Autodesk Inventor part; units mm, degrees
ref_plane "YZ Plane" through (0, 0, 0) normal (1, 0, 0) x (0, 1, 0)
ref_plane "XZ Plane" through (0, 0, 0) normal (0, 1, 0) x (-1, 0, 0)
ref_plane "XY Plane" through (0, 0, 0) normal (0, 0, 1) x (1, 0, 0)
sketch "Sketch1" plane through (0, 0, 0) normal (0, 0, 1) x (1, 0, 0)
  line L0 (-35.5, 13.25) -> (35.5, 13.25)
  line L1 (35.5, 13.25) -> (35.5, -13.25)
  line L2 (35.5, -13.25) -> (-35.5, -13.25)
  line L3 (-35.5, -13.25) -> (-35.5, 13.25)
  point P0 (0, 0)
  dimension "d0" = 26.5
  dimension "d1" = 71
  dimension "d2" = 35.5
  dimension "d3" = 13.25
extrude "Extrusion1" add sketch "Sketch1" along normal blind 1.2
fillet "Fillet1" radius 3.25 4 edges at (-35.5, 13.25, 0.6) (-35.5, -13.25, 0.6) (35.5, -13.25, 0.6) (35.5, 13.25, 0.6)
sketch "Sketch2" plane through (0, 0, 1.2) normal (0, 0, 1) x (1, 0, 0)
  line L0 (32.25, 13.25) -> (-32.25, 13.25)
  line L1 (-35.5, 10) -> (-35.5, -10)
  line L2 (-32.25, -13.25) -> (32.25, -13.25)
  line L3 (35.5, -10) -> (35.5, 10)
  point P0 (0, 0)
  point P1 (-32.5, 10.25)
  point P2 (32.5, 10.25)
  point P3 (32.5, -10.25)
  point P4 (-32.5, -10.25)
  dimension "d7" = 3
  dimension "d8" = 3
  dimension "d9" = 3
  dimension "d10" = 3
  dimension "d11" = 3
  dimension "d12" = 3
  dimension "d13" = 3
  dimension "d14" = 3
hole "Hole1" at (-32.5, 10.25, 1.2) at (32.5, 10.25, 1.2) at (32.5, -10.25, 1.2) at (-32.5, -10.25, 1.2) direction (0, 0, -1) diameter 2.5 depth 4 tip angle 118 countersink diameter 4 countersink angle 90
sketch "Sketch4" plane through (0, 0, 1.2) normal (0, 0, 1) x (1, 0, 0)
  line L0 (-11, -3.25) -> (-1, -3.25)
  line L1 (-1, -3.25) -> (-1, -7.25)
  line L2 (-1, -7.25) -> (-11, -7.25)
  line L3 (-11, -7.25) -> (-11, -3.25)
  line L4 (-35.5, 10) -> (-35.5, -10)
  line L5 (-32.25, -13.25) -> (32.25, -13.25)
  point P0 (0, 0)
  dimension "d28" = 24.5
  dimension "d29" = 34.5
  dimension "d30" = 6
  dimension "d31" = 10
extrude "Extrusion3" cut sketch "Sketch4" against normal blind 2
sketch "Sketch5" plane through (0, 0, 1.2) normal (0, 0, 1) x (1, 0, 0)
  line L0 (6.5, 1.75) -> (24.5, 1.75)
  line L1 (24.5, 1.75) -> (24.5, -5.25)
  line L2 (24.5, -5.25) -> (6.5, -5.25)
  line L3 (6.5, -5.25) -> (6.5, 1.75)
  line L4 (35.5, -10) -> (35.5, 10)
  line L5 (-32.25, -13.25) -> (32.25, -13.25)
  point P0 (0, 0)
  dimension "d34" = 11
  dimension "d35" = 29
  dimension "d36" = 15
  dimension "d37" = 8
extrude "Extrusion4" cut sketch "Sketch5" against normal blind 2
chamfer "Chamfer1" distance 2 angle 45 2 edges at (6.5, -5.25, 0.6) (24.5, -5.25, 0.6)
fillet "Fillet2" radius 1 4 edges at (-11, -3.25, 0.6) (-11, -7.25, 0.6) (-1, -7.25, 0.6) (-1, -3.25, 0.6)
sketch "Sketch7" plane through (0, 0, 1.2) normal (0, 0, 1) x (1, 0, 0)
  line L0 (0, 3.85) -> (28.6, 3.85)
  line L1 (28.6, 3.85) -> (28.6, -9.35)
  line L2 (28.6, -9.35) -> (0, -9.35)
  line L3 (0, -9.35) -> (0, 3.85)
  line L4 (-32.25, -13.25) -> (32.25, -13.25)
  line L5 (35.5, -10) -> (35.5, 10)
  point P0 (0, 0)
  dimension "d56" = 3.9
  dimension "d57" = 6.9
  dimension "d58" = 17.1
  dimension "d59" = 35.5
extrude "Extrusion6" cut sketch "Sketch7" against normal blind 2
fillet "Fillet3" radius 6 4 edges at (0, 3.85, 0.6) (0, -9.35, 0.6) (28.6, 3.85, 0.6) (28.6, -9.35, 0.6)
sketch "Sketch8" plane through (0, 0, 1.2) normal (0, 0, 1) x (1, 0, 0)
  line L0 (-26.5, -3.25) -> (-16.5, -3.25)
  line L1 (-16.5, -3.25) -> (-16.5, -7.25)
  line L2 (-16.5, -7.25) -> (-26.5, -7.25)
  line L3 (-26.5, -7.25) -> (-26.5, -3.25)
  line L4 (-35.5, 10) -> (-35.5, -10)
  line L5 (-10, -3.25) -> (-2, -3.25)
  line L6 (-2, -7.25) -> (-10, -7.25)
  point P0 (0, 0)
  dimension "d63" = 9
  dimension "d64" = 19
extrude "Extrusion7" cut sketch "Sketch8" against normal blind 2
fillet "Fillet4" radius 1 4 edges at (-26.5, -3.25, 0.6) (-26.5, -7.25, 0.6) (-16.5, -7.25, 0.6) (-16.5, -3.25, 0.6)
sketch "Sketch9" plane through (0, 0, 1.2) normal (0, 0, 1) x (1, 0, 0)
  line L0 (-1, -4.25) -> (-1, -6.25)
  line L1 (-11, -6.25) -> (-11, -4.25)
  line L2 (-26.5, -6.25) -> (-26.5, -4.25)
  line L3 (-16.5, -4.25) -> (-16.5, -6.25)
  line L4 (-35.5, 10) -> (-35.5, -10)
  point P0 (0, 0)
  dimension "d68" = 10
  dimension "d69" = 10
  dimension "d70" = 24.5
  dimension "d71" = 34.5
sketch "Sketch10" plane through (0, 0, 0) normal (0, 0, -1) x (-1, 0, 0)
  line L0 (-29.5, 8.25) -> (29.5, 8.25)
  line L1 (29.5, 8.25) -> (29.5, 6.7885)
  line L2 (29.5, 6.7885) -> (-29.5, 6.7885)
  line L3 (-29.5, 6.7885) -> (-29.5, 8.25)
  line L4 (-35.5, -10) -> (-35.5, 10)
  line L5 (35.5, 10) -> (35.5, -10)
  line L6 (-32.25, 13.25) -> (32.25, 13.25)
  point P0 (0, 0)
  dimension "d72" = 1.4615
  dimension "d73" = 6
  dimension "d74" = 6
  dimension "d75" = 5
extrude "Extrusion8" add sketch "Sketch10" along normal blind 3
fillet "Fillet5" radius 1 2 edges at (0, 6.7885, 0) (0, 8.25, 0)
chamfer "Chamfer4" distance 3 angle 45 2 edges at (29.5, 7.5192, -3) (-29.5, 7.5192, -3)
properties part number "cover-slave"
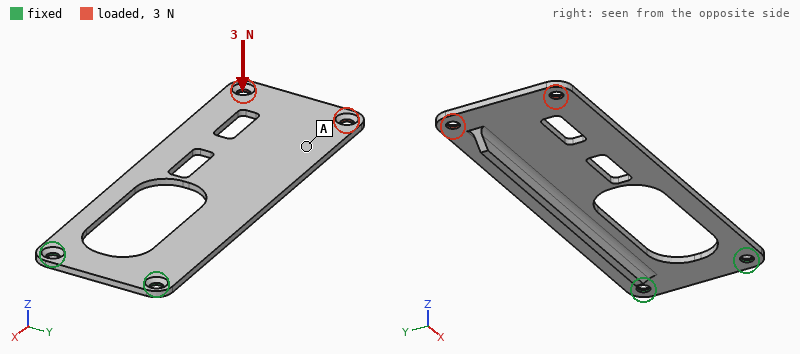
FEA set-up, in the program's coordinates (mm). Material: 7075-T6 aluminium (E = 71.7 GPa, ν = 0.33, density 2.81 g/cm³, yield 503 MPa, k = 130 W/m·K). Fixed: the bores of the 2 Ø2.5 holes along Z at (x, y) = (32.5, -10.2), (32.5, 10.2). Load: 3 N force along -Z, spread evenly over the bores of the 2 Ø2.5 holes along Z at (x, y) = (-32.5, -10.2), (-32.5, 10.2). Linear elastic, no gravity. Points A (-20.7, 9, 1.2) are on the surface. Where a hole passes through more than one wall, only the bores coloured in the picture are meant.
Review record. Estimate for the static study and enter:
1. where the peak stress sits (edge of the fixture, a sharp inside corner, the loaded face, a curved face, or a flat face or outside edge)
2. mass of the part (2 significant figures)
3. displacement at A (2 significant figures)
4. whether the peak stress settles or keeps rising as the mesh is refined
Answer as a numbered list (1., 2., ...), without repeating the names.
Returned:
1. edge of the fixture
2. 5.5 g
3. 0.50 mm
4. keeps rising
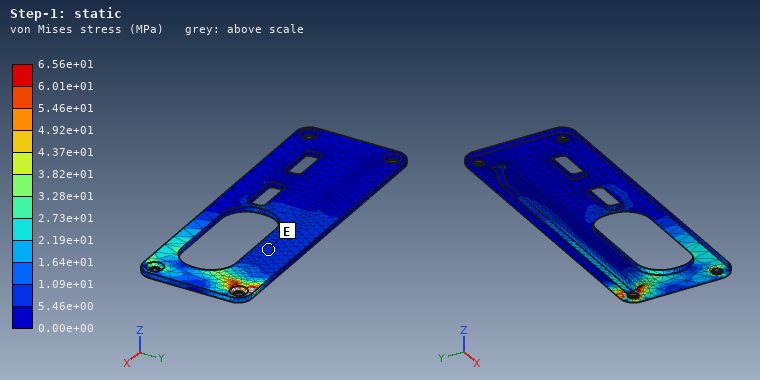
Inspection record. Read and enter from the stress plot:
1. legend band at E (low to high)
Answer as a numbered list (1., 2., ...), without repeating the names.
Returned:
1. 5.46e+00 to 1.09e+01 MPa
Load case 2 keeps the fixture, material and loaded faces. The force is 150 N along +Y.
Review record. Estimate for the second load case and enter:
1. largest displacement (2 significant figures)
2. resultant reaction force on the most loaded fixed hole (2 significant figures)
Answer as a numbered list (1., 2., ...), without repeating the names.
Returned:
1. 0.45 mm
2. 450 N
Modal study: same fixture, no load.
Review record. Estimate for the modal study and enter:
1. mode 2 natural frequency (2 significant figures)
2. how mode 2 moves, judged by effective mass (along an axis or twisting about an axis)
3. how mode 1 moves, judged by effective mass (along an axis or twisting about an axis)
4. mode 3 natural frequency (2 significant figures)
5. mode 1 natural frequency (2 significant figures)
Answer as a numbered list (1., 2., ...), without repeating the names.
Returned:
1. 1100 Hz
2. twisting about X
3. along Z
4. 2300 Hz
5. 240 Hz
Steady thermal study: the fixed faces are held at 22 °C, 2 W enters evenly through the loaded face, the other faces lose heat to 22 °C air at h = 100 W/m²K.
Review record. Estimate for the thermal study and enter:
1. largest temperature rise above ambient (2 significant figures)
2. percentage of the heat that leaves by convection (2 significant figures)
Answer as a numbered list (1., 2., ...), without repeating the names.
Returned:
1. 16 K
2. 88 %
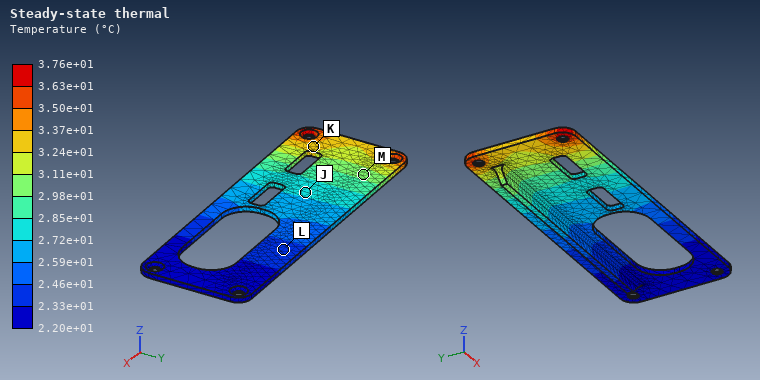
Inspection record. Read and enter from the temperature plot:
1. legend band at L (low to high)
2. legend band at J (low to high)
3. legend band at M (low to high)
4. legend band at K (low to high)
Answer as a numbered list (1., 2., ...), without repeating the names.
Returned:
1. 2.33e+01 to 2.46e+01 °C
2. 2.72e+01 to 2.85e+01 °C
3. 2.98e+01 to 3.11e+01 °C
4. 3.24e+01 to 3.37e+01 °C
